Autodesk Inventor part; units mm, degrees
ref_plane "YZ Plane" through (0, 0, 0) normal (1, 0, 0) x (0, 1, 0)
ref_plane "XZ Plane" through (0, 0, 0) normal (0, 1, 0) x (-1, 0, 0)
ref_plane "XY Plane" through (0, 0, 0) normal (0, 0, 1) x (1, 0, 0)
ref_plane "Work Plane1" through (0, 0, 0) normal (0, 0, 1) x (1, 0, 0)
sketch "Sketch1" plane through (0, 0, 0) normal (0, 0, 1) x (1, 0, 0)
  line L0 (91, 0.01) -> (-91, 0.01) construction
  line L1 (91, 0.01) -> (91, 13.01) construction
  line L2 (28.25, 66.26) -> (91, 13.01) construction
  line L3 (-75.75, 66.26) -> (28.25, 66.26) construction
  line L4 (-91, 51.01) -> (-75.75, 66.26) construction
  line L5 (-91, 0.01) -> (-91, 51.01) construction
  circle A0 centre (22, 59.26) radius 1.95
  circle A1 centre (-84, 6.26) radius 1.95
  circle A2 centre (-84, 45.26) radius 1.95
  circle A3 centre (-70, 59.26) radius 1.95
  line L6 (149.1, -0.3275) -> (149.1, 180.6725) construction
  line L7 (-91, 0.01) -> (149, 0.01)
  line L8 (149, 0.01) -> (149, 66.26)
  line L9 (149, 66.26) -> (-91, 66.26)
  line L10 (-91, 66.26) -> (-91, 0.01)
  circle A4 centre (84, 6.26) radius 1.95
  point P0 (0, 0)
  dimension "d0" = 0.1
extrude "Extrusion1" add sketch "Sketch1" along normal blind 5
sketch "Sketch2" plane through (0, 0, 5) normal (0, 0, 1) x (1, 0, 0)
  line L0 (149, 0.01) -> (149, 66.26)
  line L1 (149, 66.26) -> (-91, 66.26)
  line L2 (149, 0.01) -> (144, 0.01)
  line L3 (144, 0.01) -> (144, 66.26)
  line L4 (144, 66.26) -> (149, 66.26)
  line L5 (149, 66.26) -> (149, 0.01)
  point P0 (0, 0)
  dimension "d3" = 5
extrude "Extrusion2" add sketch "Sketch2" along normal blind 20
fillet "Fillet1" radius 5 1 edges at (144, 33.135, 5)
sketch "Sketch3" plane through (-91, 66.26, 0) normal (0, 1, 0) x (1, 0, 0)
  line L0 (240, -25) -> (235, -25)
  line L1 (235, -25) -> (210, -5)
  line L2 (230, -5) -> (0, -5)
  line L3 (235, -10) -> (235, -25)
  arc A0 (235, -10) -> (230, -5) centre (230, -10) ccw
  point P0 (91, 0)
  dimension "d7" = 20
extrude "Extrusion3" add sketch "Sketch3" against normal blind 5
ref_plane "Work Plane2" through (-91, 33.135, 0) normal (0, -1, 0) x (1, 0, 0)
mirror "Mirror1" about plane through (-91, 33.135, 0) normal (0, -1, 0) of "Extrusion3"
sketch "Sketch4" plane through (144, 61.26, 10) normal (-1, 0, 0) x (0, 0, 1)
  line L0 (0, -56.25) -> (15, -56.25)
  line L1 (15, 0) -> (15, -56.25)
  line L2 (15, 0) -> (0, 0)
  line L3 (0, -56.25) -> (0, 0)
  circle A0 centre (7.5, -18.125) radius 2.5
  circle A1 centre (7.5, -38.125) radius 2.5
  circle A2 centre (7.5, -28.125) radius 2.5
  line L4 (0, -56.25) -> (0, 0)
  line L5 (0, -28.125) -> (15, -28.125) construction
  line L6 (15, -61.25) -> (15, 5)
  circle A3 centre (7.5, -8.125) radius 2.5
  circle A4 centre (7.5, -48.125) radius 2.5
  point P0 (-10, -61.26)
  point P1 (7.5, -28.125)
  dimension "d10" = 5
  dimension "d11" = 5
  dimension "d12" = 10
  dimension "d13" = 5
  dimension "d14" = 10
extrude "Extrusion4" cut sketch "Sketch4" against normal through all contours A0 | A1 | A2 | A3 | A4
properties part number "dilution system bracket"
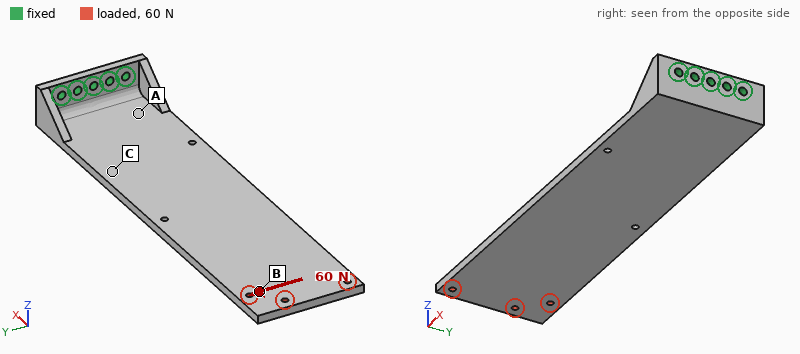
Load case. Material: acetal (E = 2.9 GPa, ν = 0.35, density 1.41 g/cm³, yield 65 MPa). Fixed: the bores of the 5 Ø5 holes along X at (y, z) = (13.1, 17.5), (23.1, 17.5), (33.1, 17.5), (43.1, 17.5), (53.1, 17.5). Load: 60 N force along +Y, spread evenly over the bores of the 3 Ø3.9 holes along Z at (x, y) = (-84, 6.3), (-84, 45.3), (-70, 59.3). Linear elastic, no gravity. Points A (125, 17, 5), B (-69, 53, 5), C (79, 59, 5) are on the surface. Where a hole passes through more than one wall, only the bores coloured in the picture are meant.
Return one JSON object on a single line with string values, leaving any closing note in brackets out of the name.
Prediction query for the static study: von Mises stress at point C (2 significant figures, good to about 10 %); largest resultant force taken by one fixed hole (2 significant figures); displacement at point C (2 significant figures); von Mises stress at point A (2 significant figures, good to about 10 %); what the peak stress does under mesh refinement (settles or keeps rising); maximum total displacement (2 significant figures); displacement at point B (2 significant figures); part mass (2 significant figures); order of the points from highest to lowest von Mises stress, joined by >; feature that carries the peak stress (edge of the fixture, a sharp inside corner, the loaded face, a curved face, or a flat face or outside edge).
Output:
{"von Mises stress at point C": "2.4 MPa", "largest resultant force taken by one fixed hole": "260 N", "displacement at point C": "0.87 mm", "von Mises stress at point A": "4.9 MPa", "what the peak stress does under mesh refinement": "keeps rising", "maximum total displacement": "2.9 mm", "displacement at point B": "2.6 mm", "part mass": "120 g", "order of the points from highest to lowest von Mises stress, joined by >": "A > C > B", "feature that carries the peak stress": "edge of the fixture"}
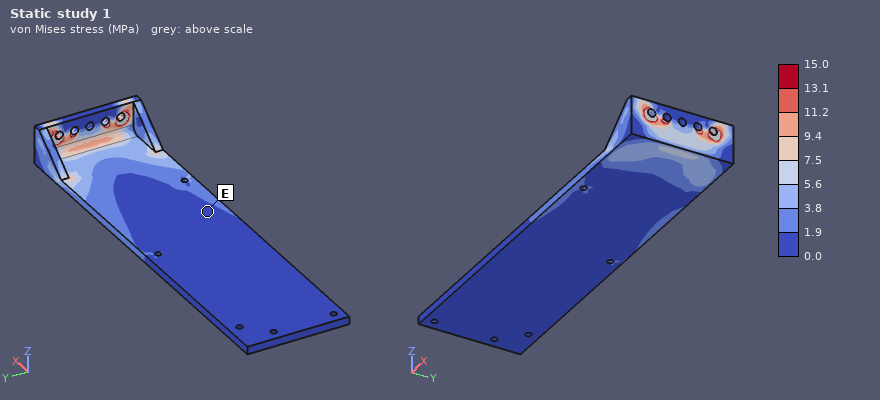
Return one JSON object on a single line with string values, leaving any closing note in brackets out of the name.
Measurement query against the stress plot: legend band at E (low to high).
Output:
{"legend band at E": "0.0 to 1.9 MPa"}
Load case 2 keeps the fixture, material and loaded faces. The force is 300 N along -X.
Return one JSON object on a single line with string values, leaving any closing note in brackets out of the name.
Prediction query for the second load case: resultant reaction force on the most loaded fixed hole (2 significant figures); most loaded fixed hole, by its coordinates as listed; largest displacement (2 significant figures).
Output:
{"resultant reaction force on the most loaded fixed hole": "87 N", "most loaded fixed hole, by its coordinates as listed": "(53.1, 17.5)", "largest displacement": "2.3 mm"}
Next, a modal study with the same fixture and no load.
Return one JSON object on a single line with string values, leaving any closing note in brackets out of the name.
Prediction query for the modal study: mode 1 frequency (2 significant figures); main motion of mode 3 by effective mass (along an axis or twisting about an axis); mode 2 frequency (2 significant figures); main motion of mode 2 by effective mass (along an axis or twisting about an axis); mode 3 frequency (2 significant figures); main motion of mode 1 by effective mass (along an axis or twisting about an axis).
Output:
{"mode 1 frequency": "22 Hz", "main motion of mode 3 by effective mass": "along Z", "mode 2 frequency": "120 Hz", "main motion of mode 2 by effective mass": "along Y", "mode 3 frequency": "140 Hz", "main motion of mode 1 by effective mass": "along Z"}
